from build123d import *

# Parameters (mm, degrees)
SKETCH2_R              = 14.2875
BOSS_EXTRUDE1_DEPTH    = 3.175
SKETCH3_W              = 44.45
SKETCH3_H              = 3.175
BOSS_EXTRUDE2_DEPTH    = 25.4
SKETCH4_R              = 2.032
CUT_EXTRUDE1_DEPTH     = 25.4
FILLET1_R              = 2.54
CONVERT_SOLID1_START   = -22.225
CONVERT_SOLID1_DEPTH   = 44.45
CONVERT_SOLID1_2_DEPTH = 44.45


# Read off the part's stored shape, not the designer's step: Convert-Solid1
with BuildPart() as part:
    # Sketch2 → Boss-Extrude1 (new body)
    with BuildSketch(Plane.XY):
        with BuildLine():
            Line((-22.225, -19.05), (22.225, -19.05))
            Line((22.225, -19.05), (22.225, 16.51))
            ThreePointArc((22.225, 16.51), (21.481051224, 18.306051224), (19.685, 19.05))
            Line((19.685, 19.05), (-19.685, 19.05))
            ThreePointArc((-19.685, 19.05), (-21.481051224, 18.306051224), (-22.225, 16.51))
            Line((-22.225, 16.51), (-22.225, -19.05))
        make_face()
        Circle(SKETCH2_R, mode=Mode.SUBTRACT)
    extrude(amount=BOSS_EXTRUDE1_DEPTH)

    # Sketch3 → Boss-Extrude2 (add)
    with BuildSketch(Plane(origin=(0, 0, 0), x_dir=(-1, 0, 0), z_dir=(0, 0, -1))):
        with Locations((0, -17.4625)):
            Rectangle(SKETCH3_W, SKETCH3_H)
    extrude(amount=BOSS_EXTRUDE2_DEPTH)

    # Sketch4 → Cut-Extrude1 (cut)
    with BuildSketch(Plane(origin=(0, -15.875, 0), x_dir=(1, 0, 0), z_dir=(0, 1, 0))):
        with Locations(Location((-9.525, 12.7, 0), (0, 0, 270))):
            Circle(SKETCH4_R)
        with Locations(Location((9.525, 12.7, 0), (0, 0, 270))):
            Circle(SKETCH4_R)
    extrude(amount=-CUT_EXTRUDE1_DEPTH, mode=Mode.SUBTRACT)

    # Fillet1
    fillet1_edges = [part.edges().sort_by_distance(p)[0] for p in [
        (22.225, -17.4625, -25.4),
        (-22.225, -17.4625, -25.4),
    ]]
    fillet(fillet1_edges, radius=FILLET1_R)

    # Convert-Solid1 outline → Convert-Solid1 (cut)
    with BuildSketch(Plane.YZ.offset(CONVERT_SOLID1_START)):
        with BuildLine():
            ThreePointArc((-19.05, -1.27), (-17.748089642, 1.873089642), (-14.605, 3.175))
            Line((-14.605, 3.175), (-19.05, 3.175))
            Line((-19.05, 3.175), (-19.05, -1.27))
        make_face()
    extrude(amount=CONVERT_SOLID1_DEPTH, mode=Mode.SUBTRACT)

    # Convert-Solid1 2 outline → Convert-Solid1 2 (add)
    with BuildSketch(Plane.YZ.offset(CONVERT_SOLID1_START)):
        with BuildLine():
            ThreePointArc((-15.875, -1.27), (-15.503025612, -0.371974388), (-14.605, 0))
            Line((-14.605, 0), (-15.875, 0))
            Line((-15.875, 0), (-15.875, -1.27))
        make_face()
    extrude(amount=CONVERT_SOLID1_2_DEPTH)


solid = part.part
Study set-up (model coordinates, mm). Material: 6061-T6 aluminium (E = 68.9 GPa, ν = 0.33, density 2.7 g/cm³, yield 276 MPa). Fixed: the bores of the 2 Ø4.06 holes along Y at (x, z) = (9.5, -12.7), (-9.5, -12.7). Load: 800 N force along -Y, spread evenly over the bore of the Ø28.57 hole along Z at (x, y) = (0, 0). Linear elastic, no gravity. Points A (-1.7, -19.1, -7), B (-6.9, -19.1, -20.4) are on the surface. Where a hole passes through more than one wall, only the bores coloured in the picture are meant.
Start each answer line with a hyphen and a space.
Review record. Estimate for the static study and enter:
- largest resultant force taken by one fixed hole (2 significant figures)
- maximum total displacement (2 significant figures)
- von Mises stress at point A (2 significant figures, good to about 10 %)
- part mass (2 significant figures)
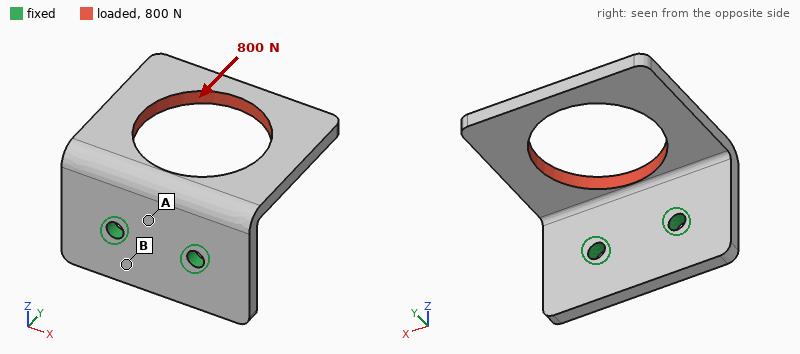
- 400 N
- 0.39 mm
- 75 MPa
- 18 g
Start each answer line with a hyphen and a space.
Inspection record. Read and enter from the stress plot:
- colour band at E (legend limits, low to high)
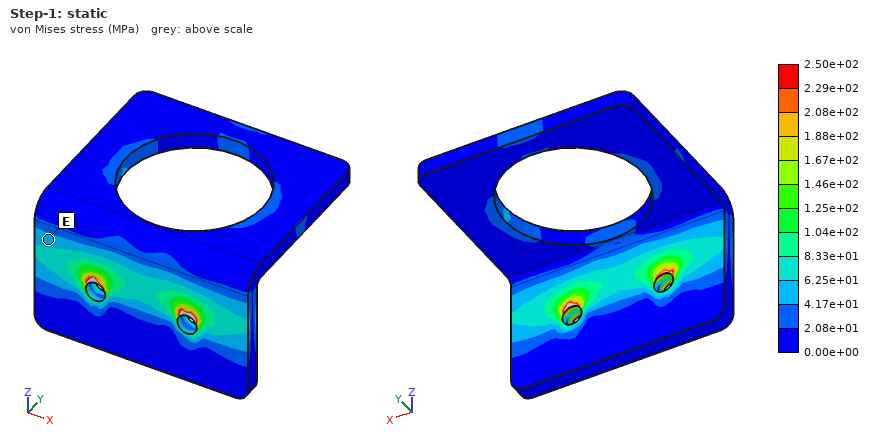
- 4.17e+01 to 6.25e+01 MPa
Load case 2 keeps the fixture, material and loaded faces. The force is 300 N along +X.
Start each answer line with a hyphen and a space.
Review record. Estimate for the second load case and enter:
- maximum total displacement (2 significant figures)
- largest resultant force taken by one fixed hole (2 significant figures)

- 0.14 mm
- 310 N
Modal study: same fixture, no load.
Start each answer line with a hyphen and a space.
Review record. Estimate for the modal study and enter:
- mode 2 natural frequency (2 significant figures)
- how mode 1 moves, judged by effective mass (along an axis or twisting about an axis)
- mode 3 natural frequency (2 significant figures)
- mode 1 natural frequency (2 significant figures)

- 2400 Hz
- along Z
- 3400 Hz
- 1200 Hz
